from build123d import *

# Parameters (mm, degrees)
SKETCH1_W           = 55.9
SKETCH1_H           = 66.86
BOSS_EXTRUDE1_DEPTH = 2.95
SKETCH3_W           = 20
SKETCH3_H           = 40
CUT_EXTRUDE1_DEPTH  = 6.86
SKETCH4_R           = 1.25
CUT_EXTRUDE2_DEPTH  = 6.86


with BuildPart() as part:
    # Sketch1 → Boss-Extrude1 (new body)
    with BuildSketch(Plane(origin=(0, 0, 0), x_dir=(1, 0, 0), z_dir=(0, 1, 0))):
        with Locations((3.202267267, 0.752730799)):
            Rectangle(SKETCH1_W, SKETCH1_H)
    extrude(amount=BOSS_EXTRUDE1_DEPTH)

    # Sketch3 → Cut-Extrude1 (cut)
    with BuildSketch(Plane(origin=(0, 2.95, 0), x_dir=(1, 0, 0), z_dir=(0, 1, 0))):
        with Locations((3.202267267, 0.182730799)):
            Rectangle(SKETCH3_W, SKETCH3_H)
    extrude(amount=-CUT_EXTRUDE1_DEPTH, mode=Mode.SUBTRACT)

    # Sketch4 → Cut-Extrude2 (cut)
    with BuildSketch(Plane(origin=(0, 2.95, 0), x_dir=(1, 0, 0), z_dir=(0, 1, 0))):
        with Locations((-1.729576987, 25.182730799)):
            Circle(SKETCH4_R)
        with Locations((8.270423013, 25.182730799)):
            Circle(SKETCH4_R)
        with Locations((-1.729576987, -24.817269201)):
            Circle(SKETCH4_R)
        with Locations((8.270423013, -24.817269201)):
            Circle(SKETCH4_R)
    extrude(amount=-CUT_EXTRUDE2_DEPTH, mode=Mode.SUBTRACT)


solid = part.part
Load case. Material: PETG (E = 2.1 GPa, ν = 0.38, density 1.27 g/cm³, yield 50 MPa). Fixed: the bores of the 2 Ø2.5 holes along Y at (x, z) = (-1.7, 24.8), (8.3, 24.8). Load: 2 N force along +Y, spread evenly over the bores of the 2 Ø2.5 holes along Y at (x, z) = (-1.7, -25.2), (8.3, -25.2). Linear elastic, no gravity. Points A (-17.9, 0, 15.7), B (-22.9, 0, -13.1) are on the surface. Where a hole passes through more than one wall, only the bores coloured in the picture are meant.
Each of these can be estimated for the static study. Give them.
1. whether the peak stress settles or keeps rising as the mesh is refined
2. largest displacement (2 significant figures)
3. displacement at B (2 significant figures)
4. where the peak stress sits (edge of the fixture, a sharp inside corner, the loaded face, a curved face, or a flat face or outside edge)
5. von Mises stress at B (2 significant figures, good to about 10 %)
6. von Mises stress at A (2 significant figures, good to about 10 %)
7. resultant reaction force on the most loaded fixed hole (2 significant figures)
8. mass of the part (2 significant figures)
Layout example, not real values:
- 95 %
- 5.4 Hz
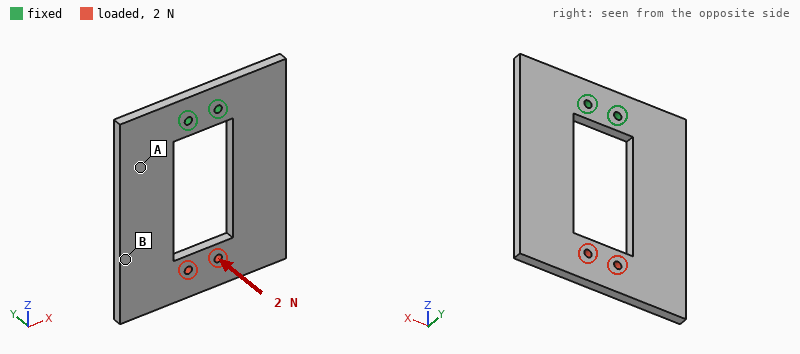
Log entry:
- keeps rising
- 1.00 mm
- 0.54 mm
- edge of the fixture
- 0.49 MPa
- 1.4 MPa
- 1.0 N
- 11 g
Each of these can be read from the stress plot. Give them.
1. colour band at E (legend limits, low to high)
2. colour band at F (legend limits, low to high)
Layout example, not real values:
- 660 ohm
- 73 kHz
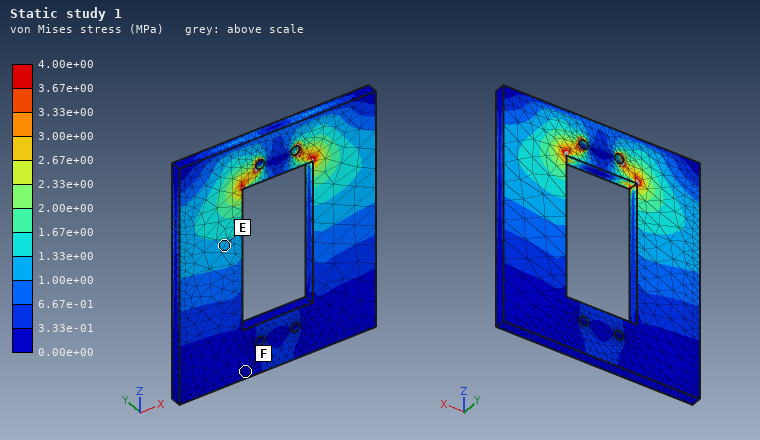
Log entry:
- 1.00e+00 to 1.33e+00 MPa
- 0.00e+00 to 3.33e-01 MPa
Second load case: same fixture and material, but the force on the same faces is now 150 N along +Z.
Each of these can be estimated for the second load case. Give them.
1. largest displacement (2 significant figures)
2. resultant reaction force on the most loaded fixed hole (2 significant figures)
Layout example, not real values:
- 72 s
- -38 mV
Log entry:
- 0.18 mm
- 78 N
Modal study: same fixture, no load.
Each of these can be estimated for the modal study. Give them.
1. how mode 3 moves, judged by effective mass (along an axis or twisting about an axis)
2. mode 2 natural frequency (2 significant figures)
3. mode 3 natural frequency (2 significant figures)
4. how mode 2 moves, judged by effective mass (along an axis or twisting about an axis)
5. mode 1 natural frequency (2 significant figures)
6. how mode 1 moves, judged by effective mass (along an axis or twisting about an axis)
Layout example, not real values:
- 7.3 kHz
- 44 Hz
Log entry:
- along X
- 260 Hz
- 510 Hz
- twisting about Z
- 120 Hz
- along Y
